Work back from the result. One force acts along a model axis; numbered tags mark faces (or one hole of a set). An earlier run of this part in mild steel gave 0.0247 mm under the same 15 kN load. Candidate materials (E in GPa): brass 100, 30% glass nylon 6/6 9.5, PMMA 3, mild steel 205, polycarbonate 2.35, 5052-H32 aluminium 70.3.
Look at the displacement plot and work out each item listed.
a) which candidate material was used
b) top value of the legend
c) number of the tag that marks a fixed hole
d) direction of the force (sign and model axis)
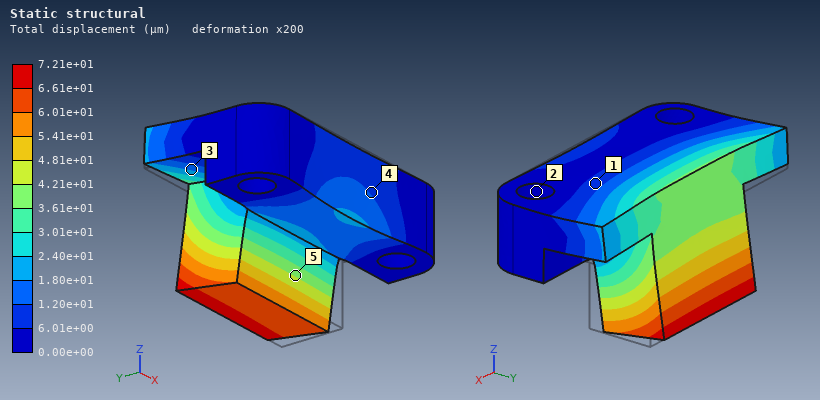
5052-H32 aluminium
7.21e+01 µm
2
+Y
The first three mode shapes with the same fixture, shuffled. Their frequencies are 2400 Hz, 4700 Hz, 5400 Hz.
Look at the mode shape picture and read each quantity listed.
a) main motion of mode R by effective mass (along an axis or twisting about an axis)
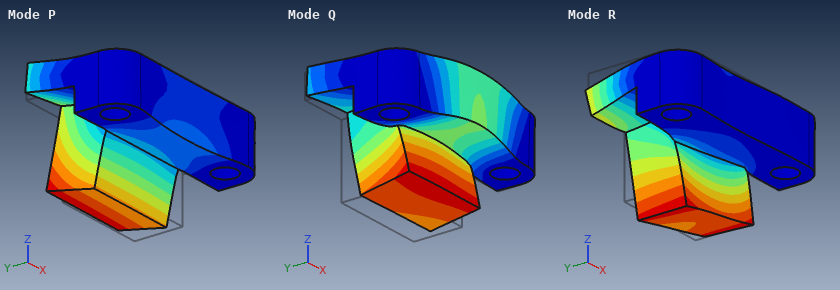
along X
